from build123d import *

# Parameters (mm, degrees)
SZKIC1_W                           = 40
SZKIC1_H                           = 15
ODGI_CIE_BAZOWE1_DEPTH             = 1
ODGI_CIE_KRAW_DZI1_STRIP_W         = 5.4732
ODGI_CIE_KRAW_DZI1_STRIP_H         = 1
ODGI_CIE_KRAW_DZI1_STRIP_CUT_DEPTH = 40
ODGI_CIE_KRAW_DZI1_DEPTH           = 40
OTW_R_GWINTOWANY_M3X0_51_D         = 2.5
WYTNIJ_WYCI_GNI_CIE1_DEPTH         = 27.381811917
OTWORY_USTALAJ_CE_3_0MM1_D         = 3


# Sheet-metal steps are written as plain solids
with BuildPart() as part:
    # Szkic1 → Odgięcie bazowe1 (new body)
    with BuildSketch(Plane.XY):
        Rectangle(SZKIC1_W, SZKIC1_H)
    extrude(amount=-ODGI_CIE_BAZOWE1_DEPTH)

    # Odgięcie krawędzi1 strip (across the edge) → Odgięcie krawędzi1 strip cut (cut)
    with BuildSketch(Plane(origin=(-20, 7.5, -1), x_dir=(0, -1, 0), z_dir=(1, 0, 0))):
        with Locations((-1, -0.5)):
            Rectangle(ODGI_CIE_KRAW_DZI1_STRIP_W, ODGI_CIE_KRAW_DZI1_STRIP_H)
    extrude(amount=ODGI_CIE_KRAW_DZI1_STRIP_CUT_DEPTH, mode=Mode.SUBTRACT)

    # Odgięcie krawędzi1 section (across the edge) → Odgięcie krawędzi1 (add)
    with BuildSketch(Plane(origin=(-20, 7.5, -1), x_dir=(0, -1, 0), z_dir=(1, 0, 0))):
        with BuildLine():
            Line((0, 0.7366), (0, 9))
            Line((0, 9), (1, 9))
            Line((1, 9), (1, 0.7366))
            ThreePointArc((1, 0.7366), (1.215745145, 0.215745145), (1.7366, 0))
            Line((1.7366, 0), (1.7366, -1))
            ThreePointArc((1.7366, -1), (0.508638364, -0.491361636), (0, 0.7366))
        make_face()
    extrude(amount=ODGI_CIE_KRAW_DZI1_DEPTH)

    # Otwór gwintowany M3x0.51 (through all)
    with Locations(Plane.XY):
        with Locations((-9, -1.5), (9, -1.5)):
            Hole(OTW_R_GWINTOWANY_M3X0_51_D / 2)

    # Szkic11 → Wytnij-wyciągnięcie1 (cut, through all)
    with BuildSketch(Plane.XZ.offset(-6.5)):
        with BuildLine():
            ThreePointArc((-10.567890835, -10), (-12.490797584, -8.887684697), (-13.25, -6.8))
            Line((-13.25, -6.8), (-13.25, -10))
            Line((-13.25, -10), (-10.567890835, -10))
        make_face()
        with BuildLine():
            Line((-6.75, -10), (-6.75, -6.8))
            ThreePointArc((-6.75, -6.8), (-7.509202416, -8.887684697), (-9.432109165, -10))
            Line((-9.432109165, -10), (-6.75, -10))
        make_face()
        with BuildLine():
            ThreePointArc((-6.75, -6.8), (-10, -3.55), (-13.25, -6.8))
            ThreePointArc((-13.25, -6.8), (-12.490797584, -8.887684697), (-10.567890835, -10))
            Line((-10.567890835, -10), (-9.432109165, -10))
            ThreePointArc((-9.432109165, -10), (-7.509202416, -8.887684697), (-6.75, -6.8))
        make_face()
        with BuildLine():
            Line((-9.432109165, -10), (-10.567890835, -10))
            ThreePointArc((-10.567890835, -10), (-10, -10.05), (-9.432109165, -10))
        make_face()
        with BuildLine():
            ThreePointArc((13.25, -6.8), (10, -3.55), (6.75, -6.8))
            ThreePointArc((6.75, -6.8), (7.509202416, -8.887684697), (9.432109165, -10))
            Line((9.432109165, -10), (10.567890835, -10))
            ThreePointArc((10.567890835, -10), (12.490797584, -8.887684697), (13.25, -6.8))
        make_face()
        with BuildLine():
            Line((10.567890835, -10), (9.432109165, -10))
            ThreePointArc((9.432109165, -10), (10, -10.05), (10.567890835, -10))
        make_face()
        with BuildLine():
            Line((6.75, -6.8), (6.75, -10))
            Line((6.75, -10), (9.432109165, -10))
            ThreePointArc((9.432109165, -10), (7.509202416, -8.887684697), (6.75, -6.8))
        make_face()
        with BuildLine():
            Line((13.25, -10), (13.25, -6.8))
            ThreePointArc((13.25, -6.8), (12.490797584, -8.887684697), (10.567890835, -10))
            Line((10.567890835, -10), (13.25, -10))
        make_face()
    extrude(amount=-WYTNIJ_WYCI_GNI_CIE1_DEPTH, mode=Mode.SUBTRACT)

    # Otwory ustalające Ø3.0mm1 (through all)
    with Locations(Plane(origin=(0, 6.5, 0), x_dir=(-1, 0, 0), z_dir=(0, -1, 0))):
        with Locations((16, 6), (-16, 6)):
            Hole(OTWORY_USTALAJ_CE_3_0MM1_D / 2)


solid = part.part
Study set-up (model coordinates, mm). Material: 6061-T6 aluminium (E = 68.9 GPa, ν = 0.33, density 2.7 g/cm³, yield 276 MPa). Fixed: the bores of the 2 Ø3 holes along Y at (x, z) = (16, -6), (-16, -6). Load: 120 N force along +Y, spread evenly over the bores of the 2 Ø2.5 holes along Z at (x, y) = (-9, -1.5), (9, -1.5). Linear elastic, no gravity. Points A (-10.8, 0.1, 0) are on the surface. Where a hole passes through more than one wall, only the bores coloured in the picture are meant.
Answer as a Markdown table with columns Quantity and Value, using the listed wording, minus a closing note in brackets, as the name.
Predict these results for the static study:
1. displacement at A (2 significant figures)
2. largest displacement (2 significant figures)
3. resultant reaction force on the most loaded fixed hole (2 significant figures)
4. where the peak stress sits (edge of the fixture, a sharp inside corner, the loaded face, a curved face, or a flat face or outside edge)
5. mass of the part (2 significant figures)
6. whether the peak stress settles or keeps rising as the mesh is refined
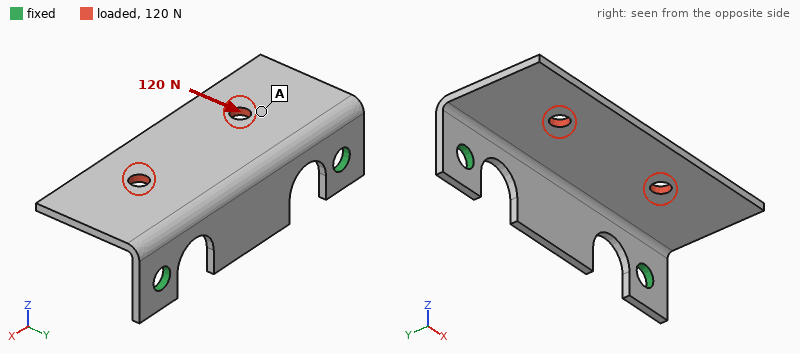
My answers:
| Quantity | Value |
|---|---|
| displacement at A | 0.096 mm |
| largest displacement | 0.18 mm |
| resultant reaction force on the most loaded fixed hole | 61 N |
| where the peak stress sits | edge of the fixture |
| mass of the part | 2.3 g |
| whether the peak stress settles or keeps rising as the mesh is refined | keeps rising |
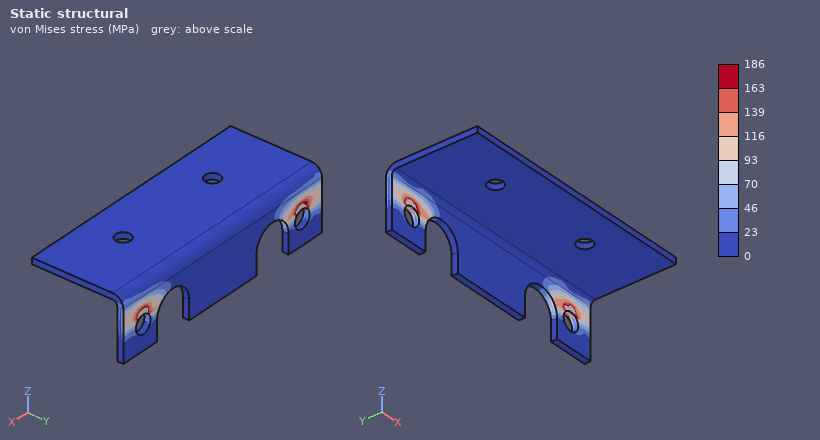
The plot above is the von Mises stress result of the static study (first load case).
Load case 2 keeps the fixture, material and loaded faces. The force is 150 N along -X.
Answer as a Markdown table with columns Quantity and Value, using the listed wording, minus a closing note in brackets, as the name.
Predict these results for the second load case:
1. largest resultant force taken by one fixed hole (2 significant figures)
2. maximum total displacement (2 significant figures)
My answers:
| Quantity | Value |
|---|---|
| largest resultant force taken by one fixed hole | 85 N |
| maximum total displacement | 63 µm |
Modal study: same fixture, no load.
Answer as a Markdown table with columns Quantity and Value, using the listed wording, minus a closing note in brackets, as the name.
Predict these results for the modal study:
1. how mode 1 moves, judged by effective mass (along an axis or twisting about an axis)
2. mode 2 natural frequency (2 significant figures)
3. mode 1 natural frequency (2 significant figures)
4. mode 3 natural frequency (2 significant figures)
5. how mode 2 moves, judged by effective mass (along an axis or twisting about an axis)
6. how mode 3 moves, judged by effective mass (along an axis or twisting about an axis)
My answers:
| Quantity | Value |
|---|---|
| how mode 1 moves, judged by effective mass | along Z |
| mode 2 natural frequency | 3800 Hz |
| mode 1 natural frequency | 1900 Hz |
| mode 3 natural frequency | 6100 Hz |
| how mode 2 moves, judged by effective mass | twisting about Y |
| how mode 3 moves, judged by effective mass | along Y |
